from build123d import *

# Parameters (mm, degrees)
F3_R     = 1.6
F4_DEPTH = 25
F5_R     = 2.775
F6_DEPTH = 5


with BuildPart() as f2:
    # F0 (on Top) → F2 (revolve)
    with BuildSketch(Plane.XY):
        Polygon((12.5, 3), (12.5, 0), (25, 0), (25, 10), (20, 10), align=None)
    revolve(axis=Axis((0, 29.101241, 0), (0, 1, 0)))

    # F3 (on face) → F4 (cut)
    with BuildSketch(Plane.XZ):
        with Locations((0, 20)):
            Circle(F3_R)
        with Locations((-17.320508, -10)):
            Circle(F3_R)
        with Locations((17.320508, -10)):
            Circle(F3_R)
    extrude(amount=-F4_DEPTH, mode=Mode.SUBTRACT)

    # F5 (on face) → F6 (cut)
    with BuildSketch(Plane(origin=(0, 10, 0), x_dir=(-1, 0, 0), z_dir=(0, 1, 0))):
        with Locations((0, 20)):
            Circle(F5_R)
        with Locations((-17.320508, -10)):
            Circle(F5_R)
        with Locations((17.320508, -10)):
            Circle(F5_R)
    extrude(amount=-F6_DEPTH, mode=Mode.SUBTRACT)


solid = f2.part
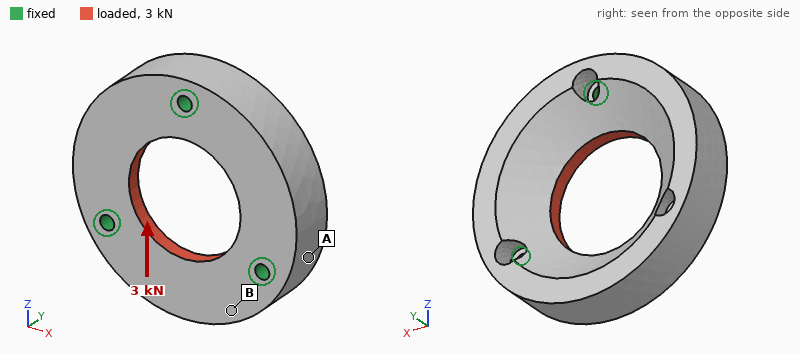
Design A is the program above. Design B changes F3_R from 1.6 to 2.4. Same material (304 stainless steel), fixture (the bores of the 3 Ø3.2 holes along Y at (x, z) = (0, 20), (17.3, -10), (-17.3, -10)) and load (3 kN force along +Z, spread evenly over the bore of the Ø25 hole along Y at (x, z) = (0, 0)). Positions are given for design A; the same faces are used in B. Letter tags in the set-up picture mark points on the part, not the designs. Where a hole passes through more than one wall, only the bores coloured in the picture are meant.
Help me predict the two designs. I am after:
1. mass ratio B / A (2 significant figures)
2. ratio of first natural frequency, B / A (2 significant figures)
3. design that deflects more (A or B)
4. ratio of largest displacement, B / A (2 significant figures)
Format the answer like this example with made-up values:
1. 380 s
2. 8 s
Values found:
1. 0.99
2. 1.2
3. A
4. 0.90
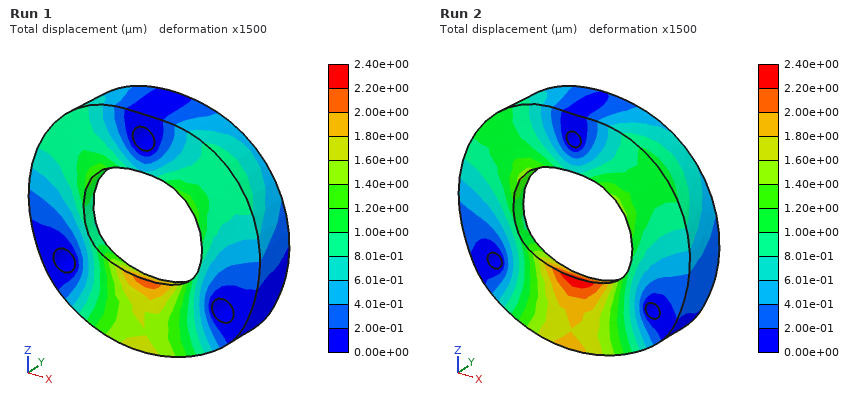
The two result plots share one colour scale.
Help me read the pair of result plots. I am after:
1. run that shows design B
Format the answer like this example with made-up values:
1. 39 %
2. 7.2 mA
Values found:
1. Run 1
